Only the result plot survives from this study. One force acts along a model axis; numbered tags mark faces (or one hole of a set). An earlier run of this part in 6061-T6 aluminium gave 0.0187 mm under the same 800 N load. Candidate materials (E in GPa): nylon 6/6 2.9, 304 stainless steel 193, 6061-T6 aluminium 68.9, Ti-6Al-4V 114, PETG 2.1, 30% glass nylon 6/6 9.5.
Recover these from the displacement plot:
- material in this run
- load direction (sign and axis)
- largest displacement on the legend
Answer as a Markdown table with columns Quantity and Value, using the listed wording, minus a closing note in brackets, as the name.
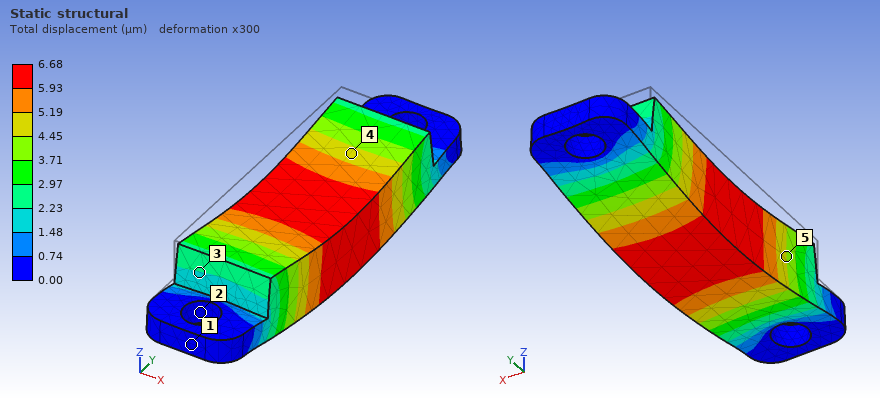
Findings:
| Quantity | Value |
|---|---|
| material in this run | 304 stainless steel |
| load direction | -Z |
| largest displacement on the legend | 6.68 µm |
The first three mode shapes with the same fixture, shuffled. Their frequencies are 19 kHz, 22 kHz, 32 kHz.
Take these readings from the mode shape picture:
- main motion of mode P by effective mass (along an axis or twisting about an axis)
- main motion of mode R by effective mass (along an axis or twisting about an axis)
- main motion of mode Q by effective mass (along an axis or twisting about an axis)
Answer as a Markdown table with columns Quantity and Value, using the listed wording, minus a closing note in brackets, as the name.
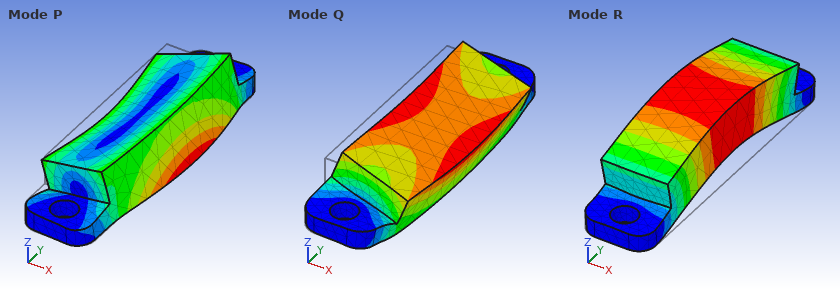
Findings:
| Quantity | Value |
|---|---|
| main motion of mode P by effective mass | along X |
| main motion of mode R by effective mass | along Z |
| main motion of mode Q by effective mass | along X |
